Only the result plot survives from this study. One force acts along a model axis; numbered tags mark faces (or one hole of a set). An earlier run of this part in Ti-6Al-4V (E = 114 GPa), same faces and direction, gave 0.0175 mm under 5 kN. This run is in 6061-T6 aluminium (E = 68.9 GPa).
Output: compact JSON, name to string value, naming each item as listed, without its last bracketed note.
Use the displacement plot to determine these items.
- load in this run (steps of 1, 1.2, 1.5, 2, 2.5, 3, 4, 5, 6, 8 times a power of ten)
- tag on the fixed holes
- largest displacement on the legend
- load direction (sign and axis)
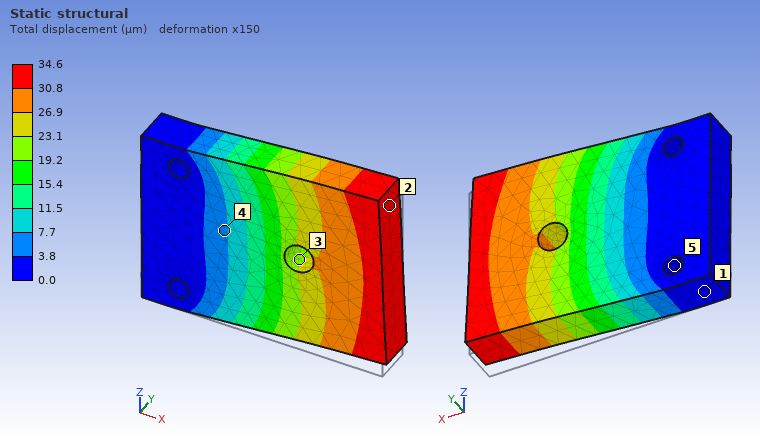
{"load in this run": "6 kN", "tag on the fixed holes": "5", "largest displacement on the legend": "34.6 µm", "load direction": "+Z"}
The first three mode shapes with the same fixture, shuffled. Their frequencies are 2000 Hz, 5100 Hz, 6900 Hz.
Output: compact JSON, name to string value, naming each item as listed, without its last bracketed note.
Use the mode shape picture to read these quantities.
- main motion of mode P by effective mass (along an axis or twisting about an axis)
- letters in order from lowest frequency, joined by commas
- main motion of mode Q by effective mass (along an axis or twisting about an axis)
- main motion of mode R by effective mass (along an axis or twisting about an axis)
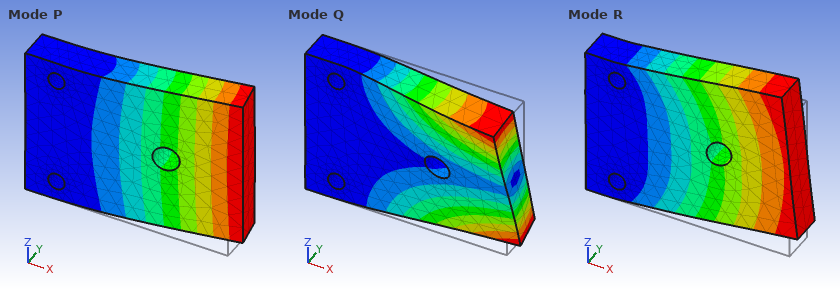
{"main motion of mode P by effective mass": "along Y", "letters in order from lowest frequency, joined by commas": "P, Q, R", "main motion of mode Q by effective mass": "twisting about X", "main motion of mode R by effective mass": "along Z"}
